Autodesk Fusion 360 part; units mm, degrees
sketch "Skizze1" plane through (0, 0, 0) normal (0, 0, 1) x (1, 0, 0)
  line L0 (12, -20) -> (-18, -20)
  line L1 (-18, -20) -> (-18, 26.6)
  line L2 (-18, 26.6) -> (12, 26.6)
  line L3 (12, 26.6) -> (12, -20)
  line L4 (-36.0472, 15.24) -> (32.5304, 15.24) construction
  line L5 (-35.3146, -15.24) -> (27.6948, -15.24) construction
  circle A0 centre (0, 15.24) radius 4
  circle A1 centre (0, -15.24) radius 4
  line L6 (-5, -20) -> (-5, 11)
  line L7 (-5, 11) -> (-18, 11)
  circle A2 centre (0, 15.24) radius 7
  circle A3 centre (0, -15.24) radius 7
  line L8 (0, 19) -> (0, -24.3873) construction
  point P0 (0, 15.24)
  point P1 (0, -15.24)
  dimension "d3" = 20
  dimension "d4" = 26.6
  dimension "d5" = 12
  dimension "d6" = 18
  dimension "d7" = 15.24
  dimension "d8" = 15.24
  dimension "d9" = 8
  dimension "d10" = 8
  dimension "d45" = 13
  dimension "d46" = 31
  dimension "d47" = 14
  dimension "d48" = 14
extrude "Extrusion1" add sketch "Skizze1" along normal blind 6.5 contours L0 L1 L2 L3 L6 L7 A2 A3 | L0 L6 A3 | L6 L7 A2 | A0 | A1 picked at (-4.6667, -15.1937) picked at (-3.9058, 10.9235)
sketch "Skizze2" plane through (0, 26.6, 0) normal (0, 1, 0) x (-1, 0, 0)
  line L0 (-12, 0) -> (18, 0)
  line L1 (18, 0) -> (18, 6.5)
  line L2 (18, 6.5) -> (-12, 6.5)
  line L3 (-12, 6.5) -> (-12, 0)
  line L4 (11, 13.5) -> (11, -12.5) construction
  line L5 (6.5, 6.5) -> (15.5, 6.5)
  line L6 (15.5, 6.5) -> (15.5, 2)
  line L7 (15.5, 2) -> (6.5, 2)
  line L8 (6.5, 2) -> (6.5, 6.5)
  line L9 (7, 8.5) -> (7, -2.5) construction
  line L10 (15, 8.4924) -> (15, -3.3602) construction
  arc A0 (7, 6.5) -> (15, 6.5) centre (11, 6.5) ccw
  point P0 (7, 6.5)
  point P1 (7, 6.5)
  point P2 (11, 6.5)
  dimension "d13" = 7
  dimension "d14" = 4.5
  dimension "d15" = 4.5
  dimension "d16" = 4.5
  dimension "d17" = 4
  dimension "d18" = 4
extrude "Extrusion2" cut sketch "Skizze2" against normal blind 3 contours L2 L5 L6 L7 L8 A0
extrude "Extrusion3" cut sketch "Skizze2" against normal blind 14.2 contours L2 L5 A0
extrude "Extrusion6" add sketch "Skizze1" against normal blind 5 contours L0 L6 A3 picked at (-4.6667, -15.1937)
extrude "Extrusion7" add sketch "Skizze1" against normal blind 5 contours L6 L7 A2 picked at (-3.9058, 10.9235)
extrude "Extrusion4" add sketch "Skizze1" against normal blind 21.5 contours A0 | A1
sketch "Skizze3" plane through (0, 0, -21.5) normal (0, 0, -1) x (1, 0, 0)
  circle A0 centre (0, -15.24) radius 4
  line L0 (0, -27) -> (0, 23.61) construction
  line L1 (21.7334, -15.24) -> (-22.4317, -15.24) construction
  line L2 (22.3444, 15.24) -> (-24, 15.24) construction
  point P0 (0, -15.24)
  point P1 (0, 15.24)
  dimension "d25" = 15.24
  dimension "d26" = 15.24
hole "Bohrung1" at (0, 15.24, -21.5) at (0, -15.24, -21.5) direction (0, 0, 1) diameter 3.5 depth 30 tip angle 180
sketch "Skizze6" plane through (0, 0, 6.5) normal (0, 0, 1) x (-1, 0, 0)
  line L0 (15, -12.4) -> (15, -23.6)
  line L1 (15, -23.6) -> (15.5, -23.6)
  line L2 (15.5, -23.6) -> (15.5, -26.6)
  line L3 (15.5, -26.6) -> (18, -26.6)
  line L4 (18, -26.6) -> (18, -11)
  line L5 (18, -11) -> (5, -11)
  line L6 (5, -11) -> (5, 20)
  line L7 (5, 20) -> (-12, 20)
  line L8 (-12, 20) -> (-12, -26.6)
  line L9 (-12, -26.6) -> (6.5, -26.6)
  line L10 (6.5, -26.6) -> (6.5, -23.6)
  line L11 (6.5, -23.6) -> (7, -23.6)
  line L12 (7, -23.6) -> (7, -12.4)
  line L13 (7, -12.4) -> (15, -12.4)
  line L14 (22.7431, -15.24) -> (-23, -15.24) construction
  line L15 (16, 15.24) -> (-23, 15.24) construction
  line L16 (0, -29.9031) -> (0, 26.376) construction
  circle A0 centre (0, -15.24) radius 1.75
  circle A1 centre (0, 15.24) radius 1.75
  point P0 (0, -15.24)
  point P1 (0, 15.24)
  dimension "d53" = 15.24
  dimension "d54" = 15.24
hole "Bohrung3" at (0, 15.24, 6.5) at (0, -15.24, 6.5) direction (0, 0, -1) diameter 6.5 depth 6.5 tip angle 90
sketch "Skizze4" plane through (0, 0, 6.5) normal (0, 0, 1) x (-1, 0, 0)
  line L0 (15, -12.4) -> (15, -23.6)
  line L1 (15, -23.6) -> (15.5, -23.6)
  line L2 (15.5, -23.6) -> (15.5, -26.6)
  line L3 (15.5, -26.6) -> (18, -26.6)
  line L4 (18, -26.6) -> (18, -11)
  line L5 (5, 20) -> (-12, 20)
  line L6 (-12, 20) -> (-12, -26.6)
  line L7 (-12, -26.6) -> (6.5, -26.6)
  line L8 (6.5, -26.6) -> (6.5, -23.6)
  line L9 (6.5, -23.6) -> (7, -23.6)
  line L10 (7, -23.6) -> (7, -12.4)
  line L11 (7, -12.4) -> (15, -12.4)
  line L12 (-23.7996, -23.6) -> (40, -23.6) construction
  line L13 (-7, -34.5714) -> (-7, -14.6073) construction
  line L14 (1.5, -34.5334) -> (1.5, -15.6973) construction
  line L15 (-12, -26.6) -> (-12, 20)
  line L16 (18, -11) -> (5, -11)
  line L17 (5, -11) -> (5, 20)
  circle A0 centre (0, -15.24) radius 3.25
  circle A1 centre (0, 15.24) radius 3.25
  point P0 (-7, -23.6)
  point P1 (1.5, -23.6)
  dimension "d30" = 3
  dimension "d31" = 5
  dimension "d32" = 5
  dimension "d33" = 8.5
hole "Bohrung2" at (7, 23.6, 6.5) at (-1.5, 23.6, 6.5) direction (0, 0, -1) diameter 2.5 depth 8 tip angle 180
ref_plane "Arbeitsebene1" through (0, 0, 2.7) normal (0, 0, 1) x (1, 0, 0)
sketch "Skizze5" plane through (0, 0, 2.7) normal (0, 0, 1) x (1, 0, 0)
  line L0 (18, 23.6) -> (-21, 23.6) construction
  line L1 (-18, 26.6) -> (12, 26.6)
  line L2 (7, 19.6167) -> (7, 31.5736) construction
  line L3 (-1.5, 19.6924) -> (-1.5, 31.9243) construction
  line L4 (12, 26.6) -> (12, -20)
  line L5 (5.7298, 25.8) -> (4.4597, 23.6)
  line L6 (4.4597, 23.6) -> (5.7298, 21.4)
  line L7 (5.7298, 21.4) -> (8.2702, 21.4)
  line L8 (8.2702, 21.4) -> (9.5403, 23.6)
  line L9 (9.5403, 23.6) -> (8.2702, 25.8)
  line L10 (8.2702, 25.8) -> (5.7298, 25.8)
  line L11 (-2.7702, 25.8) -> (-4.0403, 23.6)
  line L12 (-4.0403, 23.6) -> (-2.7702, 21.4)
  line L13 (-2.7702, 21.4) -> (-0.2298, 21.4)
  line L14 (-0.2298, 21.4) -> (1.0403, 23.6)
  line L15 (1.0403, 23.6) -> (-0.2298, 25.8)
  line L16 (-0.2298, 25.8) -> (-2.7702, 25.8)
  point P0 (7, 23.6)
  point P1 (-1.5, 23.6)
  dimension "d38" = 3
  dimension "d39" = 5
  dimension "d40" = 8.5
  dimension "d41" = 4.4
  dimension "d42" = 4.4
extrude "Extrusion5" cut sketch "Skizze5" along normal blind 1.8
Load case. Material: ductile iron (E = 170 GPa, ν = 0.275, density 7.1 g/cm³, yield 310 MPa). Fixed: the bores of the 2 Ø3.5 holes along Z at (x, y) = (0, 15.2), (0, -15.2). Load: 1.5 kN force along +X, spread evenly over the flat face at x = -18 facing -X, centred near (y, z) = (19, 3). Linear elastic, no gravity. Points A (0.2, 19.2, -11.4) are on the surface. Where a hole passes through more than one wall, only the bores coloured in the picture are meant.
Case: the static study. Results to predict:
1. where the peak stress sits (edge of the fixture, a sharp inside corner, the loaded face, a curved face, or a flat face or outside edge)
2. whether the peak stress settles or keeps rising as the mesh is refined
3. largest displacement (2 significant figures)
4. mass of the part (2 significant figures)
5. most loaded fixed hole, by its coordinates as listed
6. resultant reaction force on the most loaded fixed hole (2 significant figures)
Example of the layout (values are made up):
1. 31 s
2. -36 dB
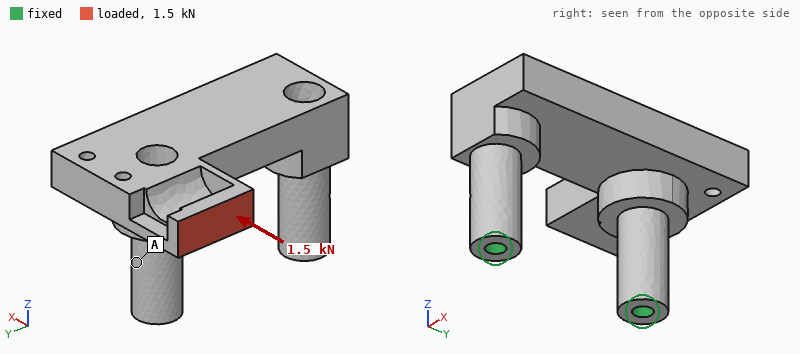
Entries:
1. edge of the fixture
2. keeps rising
3. 48 µm
4. 58 g
5. (0, 15.2)
6. 1.5 kN
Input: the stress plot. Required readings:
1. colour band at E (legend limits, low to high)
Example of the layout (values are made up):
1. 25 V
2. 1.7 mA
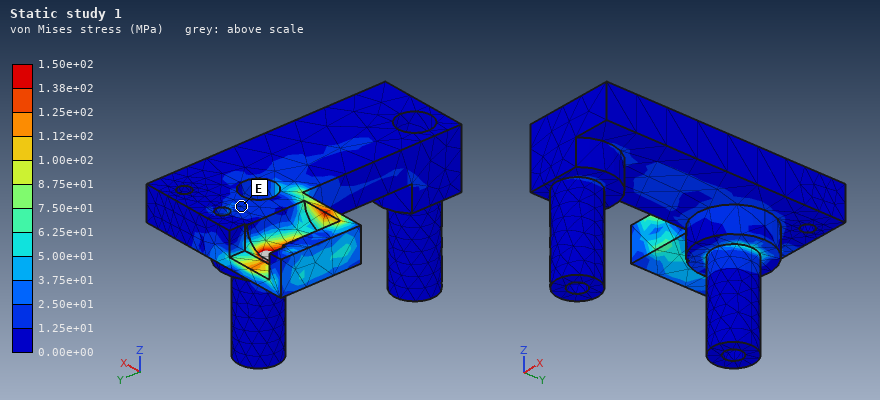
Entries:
1. 1.25e+01 to 2.50e+01 MPa
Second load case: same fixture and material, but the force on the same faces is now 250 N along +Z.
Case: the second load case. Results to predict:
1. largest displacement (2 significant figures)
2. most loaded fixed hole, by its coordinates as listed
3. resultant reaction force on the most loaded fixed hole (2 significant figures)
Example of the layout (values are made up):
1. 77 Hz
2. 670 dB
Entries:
1. 30 µm
2. (0, 15.2)
3. 270 N
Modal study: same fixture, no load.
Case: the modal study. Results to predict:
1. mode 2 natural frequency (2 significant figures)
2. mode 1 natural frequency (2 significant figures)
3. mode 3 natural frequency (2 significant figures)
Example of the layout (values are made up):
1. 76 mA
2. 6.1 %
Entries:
1. 15 kHz
2. 9800 Hz
3. 16 kHz
